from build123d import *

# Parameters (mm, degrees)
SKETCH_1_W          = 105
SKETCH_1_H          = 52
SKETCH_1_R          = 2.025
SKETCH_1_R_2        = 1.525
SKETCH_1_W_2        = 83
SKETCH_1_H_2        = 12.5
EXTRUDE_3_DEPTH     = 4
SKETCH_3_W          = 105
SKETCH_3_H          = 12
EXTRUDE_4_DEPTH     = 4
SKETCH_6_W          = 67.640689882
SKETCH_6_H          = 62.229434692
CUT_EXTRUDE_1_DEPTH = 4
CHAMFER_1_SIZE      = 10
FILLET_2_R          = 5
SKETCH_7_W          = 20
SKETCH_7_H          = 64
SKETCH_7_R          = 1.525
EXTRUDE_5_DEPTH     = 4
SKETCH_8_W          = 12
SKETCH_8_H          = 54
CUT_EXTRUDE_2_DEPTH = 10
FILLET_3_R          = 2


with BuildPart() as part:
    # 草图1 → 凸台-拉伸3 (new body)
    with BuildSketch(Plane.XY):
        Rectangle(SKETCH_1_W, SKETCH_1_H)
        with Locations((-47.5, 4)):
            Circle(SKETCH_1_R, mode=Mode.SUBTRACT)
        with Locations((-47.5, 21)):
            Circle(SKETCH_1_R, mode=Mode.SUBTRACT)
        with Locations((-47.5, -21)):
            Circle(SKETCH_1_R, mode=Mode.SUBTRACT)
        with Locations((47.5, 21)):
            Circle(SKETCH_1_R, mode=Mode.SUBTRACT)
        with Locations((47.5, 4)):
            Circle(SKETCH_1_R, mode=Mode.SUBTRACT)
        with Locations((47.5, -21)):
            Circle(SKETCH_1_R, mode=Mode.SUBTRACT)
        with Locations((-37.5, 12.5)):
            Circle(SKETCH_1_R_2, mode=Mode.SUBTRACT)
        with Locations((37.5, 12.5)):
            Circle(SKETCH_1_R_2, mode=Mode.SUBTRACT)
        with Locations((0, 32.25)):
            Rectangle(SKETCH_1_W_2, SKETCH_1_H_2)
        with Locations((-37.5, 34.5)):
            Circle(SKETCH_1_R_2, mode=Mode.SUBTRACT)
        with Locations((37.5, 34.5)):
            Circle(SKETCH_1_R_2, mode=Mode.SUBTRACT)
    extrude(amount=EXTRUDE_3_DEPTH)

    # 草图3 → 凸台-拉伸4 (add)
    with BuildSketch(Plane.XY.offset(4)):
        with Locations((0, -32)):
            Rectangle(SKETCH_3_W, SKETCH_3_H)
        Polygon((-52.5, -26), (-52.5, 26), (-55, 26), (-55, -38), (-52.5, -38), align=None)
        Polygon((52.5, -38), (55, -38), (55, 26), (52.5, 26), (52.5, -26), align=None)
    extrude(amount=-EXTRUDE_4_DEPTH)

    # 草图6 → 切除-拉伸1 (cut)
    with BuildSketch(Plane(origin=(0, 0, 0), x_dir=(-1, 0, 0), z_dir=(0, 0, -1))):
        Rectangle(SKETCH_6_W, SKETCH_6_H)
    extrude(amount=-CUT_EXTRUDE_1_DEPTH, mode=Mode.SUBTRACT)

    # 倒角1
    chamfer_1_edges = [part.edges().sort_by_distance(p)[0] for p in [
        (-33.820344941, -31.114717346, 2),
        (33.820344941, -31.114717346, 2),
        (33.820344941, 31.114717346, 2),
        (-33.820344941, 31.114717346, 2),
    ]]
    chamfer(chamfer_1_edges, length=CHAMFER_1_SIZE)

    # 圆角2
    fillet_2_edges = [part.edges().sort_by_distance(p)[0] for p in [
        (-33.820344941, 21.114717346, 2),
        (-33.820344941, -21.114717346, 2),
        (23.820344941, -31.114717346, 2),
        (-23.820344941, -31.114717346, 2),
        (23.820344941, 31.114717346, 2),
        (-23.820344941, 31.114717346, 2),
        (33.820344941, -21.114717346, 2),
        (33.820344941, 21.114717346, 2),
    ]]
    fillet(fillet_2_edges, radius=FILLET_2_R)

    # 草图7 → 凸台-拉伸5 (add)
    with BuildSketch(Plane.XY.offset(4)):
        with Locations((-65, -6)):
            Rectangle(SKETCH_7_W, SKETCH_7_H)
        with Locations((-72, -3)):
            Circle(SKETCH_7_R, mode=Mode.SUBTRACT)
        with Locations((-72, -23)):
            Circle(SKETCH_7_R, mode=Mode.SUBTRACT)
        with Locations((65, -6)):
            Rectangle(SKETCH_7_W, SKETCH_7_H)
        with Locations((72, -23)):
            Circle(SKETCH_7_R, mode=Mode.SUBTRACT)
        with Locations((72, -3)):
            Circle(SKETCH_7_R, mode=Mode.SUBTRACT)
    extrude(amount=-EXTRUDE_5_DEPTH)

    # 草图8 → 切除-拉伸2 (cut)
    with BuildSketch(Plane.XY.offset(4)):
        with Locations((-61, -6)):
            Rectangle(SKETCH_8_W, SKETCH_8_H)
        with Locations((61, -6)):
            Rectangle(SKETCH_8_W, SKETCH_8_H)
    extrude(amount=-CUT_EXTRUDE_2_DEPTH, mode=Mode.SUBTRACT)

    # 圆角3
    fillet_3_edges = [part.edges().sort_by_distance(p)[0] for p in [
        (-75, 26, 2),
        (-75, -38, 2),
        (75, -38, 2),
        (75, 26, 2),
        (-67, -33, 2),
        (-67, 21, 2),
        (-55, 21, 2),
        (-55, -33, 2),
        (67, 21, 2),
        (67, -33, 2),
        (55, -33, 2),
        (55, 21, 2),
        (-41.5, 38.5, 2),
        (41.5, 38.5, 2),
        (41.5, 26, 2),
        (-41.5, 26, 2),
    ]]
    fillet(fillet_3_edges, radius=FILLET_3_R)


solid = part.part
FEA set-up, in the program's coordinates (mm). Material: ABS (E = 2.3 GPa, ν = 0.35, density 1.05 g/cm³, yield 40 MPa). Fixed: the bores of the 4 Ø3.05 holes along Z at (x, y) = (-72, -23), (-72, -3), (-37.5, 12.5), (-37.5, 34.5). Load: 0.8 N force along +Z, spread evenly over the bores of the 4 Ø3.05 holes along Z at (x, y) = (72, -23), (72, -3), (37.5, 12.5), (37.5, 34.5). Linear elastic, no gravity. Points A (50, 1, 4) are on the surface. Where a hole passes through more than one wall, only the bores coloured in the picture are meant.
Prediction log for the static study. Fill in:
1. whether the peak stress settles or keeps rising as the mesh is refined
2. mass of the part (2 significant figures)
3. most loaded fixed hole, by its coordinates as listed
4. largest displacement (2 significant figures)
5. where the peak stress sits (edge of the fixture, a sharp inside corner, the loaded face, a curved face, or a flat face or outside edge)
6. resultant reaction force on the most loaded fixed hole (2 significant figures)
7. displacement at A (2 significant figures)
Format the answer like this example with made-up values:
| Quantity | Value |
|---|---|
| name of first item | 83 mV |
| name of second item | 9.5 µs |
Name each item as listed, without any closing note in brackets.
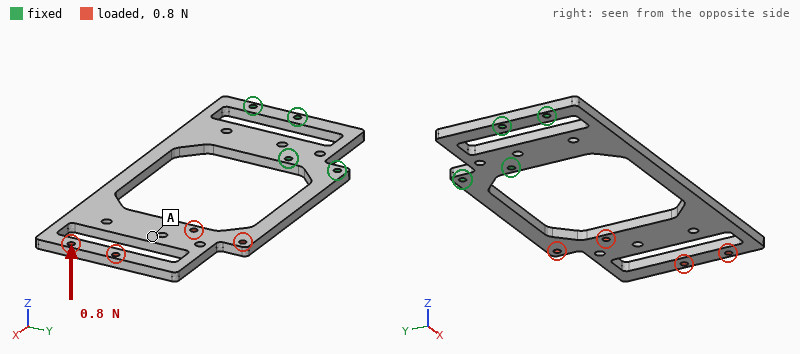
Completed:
| Quantity | Value |
|---|---|
| whether the peak stress settles or keeps rising as the mesh is refined | keeps rising |
| mass of the part | 22 g |
| most loaded fixed hole, by its coordinates as listed | (-37.5, 34.5) |
| largest displacement | 1.7 mm |
| where the peak stress sits | edge of the fixture |
| resultant reaction force on the most loaded fixed hole | 0.77 N |
| displacement at A | 1.1 mm |
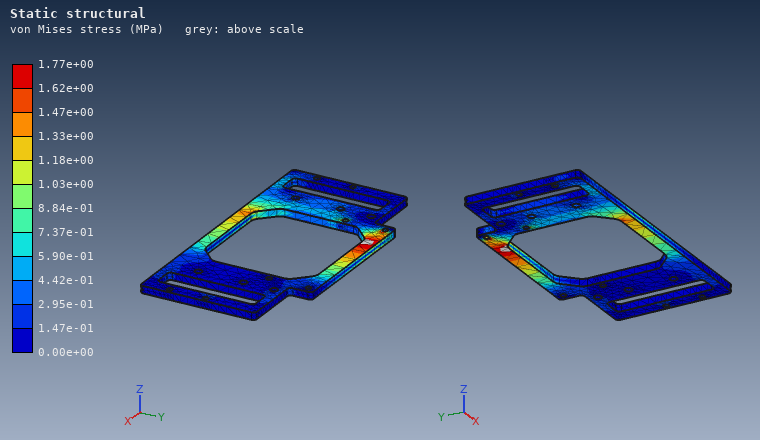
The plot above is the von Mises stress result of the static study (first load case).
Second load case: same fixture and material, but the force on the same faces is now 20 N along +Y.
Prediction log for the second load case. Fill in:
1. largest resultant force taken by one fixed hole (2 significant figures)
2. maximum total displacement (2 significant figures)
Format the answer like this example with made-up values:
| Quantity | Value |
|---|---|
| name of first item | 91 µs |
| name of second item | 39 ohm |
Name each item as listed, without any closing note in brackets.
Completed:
| Quantity | Value |
|---|---|
| largest resultant force taken by one fixed hole | 38 N |
| maximum total displacement | 0.79 mm |
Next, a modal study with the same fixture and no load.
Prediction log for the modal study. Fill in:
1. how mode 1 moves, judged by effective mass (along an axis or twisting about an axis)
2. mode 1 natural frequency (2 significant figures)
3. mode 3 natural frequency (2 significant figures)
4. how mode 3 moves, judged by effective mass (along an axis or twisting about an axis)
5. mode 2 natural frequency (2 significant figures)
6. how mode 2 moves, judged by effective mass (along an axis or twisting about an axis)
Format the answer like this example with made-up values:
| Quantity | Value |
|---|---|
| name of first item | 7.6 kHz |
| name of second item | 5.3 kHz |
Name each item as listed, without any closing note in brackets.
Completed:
| Quantity | Value |
|---|---|
| how mode 1 moves, judged by effective mass | along Z |
| mode 1 natural frequency | 43 Hz |
| mode 3 natural frequency | 260 Hz |
| how mode 3 moves, judged by effective mass | along Y |
| mode 2 natural frequency | 160 Hz |
| how mode 2 moves, judged by effective mass | twisting about X |
